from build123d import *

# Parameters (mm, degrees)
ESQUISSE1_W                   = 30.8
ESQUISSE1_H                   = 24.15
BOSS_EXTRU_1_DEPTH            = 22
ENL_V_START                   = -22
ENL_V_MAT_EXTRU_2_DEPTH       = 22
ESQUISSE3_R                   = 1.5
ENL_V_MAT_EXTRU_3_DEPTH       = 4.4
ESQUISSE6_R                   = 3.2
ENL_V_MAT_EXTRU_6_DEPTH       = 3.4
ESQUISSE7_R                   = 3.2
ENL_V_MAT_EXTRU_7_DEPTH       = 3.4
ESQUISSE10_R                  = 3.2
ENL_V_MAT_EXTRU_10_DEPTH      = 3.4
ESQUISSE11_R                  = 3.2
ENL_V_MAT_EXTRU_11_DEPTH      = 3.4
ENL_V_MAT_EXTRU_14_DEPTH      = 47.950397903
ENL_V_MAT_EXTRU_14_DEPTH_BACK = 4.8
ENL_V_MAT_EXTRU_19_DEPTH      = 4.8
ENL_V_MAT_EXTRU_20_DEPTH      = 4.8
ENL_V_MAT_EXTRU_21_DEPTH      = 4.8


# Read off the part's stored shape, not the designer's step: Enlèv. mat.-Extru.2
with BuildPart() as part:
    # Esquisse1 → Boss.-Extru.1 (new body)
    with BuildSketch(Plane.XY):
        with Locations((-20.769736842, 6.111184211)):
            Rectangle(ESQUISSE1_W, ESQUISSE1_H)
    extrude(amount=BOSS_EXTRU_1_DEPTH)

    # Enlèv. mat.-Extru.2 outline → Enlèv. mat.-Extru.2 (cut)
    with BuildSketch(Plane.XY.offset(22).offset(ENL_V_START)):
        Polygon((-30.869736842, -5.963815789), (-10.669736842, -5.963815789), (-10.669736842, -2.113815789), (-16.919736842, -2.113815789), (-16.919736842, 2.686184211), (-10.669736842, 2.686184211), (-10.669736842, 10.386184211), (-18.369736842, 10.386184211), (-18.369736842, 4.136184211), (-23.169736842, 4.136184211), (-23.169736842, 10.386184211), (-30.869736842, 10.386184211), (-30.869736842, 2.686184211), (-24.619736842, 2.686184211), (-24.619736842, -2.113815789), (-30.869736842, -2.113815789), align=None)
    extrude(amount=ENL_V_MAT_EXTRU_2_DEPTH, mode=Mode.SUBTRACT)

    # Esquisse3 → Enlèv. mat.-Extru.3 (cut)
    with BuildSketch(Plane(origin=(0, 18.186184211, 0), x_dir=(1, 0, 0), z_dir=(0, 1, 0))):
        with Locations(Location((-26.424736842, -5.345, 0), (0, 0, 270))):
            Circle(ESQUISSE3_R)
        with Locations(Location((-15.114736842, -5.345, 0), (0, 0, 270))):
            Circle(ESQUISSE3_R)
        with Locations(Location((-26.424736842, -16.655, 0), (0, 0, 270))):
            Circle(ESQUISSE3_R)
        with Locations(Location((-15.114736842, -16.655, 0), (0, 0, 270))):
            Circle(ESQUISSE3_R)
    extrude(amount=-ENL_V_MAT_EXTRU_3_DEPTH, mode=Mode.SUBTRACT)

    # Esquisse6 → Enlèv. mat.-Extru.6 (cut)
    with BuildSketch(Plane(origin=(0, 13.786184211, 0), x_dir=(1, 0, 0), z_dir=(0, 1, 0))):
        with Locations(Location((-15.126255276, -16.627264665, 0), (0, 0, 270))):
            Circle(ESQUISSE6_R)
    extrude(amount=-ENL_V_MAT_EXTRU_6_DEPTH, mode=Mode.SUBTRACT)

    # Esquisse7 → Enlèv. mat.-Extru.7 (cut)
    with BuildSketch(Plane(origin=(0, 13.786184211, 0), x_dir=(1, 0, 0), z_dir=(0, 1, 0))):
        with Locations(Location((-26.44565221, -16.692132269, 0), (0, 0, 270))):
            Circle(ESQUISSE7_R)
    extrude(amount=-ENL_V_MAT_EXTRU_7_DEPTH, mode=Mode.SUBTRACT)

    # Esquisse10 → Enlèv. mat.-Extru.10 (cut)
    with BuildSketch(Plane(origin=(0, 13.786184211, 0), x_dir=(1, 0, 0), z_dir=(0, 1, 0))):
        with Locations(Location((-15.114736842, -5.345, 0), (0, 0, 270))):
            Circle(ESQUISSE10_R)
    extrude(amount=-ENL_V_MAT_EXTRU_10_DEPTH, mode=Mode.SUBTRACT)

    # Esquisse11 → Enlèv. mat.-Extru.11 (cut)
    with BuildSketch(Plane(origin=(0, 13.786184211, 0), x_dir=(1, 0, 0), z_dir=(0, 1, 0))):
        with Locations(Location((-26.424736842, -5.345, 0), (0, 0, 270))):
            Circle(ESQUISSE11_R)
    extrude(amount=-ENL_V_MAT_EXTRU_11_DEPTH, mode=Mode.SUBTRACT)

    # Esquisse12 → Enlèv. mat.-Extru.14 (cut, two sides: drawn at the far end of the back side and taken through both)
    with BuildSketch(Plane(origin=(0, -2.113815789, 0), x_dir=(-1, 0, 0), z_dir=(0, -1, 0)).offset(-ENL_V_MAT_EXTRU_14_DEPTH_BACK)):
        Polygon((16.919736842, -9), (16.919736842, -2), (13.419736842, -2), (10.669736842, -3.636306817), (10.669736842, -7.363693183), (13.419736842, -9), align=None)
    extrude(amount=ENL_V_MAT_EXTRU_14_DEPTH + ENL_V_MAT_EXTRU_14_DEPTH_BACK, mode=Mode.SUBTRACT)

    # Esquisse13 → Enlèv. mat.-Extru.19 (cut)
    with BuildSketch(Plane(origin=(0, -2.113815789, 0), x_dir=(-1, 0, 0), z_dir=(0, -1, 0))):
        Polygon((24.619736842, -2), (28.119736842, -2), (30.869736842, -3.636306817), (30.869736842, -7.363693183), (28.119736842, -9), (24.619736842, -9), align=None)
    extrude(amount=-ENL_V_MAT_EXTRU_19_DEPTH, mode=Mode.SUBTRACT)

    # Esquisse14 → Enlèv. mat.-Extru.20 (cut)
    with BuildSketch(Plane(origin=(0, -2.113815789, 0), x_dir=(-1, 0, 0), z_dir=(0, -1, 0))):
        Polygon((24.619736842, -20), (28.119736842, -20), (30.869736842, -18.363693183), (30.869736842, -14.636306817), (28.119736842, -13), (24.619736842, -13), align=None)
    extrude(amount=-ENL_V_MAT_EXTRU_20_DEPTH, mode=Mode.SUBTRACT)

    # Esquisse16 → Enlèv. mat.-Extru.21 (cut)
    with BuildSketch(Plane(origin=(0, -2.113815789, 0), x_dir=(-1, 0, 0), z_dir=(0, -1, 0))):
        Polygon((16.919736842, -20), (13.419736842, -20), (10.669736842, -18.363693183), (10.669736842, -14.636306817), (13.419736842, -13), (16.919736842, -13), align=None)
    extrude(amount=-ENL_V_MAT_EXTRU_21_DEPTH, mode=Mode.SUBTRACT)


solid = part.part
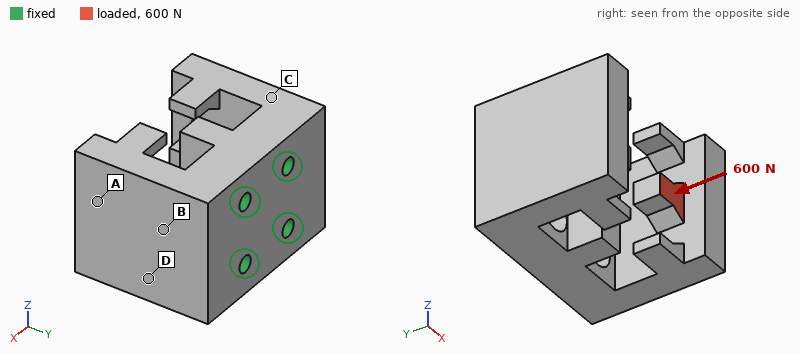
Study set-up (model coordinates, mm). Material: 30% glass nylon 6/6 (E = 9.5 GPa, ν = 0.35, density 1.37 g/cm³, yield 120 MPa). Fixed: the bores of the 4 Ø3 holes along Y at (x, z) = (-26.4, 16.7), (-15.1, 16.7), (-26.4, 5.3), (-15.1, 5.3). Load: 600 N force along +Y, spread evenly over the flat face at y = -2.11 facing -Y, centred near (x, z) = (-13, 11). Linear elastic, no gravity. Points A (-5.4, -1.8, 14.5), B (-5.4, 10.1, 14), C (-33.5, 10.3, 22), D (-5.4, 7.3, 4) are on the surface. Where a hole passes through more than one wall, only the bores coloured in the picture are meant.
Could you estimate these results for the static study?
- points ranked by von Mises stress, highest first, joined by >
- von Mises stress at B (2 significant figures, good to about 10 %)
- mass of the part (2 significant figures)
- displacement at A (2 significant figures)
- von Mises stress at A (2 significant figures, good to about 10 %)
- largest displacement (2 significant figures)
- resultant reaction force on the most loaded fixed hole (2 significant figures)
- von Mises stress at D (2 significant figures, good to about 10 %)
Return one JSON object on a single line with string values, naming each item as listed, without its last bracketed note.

{"points ranked by von Mises stress, highest first, joined by >": "D > B > A > C", "von Mises stress at B": "20 MPa", "mass of the part": "13 g", "displacement at A": "0.13 mm", "von Mises stress at A": "9.3 MPa", "largest displacement": "0.28 mm", "resultant reaction force on the most loaded fixed hole": "310 N", "von Mises stress at D": "24 MPa"}
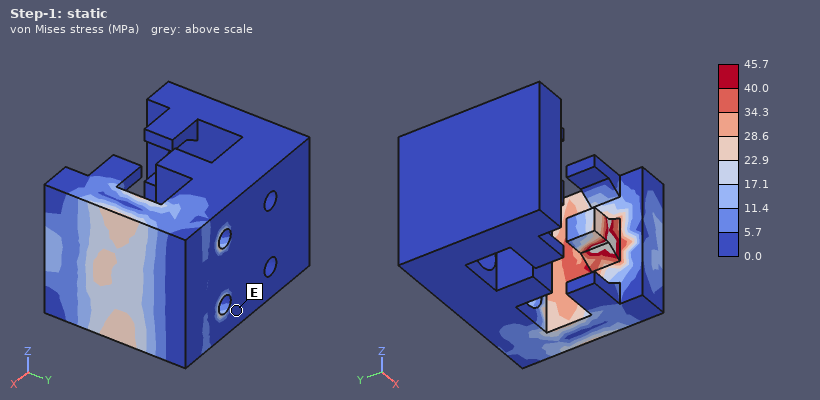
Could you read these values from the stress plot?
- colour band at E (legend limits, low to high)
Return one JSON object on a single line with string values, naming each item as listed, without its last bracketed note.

{"colour band at E": "0.0 to 5.7 MPa"}
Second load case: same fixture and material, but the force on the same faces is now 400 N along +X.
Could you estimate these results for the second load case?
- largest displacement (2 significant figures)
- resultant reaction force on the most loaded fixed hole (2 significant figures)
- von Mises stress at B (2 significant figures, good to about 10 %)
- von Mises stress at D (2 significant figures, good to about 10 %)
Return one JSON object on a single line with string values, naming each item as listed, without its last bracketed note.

{"largest displacement": "0.45 mm", "resultant reaction force on the most loaded fixed hole": "280 N", "von Mises stress at B": "38 MPa", "von Mises stress at D": "35 MPa"}
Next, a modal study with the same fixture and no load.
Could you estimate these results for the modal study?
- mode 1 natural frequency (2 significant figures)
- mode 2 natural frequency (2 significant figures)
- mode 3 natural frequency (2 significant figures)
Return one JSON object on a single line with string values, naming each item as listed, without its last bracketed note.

{"mode 1 natural frequency": "3900 Hz", "mode 2 natural frequency": "4000 Hz", "mode 3 natural frequency": "6400 Hz"}
